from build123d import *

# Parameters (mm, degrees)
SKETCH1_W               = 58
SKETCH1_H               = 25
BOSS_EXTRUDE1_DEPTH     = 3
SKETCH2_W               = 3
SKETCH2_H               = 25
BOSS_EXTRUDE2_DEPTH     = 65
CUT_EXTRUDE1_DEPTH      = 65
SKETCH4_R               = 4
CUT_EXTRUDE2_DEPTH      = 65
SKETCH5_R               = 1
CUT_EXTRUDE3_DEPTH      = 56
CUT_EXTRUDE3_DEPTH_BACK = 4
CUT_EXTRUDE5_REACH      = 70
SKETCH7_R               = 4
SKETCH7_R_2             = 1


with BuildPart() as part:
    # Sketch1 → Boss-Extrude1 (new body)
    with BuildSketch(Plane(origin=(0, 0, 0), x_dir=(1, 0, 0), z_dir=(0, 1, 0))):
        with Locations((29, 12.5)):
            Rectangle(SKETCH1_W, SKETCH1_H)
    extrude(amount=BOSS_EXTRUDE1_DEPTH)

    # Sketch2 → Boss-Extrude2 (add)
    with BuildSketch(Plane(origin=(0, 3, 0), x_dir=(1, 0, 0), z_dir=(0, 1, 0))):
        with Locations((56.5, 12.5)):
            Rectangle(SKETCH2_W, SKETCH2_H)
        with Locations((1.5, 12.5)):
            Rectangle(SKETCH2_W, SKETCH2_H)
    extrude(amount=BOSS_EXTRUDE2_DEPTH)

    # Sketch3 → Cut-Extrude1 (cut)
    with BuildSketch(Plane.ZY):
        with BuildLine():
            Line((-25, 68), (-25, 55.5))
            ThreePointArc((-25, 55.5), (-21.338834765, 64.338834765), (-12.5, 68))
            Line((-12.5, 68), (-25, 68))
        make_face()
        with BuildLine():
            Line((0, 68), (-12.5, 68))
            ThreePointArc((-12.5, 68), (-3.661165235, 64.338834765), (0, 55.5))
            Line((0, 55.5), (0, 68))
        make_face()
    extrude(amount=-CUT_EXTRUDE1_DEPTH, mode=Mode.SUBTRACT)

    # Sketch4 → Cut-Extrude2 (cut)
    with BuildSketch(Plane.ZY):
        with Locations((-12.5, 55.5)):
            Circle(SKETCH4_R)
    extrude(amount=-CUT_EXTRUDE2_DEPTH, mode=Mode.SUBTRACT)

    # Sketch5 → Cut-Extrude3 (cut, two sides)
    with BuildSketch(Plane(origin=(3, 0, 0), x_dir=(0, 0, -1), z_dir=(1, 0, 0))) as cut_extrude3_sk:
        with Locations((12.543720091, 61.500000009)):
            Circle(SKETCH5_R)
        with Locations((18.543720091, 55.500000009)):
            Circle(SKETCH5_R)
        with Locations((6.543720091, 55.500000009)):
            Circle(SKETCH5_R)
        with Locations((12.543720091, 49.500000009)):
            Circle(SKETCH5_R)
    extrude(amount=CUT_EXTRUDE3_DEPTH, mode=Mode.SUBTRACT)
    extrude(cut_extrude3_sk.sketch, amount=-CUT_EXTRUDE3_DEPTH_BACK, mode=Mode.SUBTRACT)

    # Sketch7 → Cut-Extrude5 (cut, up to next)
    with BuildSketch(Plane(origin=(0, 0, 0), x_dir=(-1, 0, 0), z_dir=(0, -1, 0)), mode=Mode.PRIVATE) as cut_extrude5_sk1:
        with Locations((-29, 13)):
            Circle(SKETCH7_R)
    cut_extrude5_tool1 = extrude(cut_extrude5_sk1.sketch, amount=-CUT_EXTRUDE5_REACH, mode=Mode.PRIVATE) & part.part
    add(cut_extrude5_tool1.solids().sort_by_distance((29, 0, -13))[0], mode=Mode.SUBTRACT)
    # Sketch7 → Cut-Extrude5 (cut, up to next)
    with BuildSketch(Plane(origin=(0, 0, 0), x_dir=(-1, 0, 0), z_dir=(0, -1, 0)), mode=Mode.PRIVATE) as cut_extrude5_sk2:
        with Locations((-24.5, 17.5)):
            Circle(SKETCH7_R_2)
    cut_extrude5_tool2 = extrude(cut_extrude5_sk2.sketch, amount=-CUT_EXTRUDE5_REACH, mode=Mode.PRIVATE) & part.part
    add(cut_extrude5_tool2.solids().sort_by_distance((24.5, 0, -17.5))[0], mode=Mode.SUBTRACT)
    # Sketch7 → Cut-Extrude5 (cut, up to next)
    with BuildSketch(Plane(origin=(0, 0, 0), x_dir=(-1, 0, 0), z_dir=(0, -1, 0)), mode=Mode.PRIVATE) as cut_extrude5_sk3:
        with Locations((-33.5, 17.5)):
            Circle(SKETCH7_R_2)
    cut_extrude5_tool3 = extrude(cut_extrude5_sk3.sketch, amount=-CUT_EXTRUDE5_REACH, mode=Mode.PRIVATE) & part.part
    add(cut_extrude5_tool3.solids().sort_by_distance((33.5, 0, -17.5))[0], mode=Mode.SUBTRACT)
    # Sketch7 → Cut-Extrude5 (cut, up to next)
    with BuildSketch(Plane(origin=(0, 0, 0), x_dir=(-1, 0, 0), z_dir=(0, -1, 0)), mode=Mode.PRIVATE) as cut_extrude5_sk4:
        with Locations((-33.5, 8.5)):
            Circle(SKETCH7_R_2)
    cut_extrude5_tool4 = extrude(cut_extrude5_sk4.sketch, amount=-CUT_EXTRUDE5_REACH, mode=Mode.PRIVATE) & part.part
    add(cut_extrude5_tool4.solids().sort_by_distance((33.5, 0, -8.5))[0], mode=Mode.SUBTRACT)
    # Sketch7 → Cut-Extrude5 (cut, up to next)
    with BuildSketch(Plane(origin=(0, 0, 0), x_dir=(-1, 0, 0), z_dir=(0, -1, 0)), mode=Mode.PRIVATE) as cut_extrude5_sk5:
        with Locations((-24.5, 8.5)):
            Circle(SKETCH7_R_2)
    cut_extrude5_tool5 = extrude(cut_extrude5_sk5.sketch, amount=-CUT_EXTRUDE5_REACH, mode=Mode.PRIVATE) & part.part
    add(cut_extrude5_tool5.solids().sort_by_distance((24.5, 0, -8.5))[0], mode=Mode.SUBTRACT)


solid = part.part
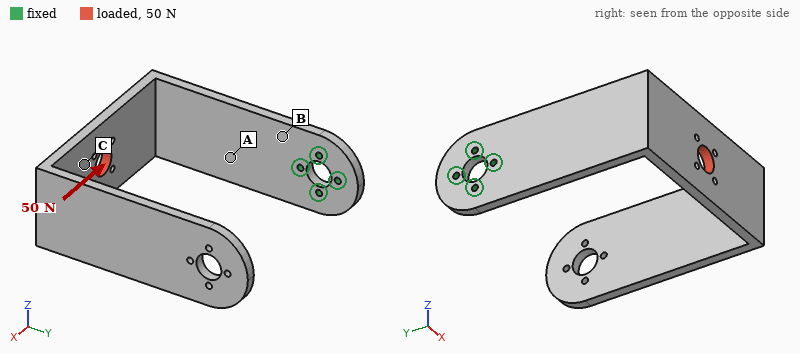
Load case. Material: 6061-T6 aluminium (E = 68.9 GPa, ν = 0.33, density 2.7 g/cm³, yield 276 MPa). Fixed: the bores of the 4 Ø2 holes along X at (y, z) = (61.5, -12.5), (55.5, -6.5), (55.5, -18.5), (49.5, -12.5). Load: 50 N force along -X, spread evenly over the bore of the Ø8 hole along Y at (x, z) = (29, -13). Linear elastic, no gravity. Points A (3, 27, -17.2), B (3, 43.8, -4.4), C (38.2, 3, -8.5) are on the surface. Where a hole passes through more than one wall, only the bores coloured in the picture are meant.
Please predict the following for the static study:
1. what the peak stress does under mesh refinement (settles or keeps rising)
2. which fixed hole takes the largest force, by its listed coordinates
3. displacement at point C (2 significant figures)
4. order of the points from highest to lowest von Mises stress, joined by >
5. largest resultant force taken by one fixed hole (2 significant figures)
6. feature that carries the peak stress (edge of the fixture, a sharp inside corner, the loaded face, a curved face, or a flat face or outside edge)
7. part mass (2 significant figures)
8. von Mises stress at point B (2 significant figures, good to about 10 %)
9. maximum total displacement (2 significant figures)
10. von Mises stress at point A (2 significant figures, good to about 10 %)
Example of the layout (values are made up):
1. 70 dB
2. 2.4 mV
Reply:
1. keeps rising
2. (49.5, -12.5)
3. 0.73 mm
4. B > A > C
5. 230 N
6. edge of the fixture
7. 35 g
8. 52 MPa
9. 1.0 mm
10. 32 MPa
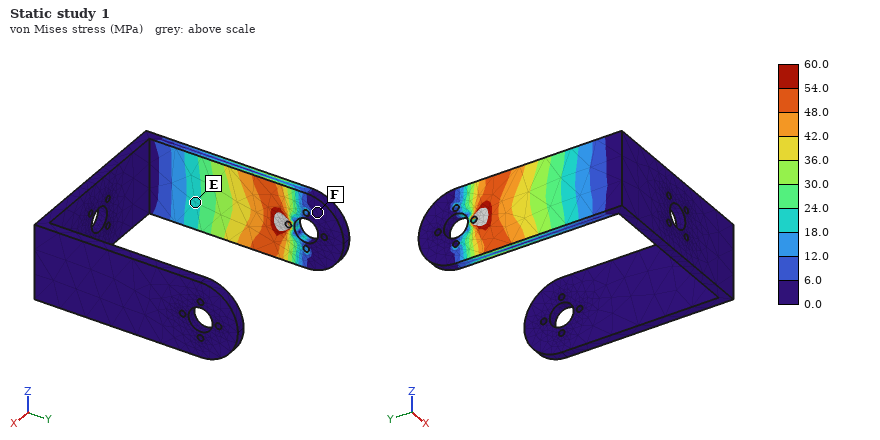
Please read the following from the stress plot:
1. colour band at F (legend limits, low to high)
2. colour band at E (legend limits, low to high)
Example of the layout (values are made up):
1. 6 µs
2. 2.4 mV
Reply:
1. 0.0 to 6.0 MPa
2. 18.0 to 24.0 MPa
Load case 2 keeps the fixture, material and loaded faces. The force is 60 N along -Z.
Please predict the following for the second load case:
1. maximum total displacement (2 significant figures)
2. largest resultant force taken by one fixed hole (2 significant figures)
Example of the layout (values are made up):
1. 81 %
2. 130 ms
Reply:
1. 0.83 mm
2. 170 N
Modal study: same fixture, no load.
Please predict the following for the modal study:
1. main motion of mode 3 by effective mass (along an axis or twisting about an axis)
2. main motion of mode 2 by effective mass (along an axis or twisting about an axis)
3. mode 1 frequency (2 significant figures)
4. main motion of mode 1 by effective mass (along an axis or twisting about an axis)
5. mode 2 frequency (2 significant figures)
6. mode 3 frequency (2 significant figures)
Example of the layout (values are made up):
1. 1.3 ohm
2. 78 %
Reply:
1. along X
2. along Z
3. 160 Hz
4. along Y
5. 220 Hz
6. 330 Hz
